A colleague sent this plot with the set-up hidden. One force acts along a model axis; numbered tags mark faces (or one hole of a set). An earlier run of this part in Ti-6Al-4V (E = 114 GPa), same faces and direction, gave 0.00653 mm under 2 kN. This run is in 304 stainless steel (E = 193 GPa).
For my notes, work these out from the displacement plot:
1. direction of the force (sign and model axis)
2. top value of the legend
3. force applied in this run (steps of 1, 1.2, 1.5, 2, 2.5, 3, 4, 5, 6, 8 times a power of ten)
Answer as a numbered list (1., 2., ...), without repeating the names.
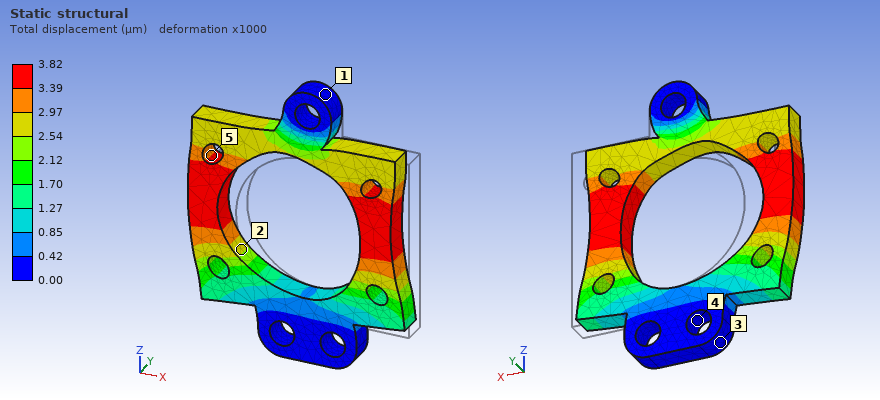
1. -X
2. 3.82 µm
3. 2 kN
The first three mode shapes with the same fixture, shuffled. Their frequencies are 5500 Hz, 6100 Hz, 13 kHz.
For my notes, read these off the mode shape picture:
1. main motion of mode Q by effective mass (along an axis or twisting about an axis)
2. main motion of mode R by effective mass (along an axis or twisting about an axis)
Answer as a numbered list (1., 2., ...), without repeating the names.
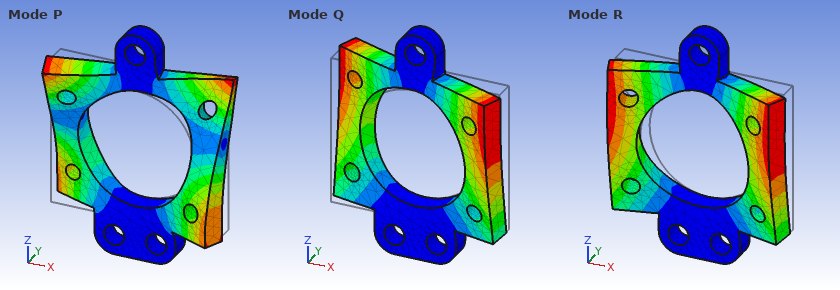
1. twisting about Z
2. along Y
